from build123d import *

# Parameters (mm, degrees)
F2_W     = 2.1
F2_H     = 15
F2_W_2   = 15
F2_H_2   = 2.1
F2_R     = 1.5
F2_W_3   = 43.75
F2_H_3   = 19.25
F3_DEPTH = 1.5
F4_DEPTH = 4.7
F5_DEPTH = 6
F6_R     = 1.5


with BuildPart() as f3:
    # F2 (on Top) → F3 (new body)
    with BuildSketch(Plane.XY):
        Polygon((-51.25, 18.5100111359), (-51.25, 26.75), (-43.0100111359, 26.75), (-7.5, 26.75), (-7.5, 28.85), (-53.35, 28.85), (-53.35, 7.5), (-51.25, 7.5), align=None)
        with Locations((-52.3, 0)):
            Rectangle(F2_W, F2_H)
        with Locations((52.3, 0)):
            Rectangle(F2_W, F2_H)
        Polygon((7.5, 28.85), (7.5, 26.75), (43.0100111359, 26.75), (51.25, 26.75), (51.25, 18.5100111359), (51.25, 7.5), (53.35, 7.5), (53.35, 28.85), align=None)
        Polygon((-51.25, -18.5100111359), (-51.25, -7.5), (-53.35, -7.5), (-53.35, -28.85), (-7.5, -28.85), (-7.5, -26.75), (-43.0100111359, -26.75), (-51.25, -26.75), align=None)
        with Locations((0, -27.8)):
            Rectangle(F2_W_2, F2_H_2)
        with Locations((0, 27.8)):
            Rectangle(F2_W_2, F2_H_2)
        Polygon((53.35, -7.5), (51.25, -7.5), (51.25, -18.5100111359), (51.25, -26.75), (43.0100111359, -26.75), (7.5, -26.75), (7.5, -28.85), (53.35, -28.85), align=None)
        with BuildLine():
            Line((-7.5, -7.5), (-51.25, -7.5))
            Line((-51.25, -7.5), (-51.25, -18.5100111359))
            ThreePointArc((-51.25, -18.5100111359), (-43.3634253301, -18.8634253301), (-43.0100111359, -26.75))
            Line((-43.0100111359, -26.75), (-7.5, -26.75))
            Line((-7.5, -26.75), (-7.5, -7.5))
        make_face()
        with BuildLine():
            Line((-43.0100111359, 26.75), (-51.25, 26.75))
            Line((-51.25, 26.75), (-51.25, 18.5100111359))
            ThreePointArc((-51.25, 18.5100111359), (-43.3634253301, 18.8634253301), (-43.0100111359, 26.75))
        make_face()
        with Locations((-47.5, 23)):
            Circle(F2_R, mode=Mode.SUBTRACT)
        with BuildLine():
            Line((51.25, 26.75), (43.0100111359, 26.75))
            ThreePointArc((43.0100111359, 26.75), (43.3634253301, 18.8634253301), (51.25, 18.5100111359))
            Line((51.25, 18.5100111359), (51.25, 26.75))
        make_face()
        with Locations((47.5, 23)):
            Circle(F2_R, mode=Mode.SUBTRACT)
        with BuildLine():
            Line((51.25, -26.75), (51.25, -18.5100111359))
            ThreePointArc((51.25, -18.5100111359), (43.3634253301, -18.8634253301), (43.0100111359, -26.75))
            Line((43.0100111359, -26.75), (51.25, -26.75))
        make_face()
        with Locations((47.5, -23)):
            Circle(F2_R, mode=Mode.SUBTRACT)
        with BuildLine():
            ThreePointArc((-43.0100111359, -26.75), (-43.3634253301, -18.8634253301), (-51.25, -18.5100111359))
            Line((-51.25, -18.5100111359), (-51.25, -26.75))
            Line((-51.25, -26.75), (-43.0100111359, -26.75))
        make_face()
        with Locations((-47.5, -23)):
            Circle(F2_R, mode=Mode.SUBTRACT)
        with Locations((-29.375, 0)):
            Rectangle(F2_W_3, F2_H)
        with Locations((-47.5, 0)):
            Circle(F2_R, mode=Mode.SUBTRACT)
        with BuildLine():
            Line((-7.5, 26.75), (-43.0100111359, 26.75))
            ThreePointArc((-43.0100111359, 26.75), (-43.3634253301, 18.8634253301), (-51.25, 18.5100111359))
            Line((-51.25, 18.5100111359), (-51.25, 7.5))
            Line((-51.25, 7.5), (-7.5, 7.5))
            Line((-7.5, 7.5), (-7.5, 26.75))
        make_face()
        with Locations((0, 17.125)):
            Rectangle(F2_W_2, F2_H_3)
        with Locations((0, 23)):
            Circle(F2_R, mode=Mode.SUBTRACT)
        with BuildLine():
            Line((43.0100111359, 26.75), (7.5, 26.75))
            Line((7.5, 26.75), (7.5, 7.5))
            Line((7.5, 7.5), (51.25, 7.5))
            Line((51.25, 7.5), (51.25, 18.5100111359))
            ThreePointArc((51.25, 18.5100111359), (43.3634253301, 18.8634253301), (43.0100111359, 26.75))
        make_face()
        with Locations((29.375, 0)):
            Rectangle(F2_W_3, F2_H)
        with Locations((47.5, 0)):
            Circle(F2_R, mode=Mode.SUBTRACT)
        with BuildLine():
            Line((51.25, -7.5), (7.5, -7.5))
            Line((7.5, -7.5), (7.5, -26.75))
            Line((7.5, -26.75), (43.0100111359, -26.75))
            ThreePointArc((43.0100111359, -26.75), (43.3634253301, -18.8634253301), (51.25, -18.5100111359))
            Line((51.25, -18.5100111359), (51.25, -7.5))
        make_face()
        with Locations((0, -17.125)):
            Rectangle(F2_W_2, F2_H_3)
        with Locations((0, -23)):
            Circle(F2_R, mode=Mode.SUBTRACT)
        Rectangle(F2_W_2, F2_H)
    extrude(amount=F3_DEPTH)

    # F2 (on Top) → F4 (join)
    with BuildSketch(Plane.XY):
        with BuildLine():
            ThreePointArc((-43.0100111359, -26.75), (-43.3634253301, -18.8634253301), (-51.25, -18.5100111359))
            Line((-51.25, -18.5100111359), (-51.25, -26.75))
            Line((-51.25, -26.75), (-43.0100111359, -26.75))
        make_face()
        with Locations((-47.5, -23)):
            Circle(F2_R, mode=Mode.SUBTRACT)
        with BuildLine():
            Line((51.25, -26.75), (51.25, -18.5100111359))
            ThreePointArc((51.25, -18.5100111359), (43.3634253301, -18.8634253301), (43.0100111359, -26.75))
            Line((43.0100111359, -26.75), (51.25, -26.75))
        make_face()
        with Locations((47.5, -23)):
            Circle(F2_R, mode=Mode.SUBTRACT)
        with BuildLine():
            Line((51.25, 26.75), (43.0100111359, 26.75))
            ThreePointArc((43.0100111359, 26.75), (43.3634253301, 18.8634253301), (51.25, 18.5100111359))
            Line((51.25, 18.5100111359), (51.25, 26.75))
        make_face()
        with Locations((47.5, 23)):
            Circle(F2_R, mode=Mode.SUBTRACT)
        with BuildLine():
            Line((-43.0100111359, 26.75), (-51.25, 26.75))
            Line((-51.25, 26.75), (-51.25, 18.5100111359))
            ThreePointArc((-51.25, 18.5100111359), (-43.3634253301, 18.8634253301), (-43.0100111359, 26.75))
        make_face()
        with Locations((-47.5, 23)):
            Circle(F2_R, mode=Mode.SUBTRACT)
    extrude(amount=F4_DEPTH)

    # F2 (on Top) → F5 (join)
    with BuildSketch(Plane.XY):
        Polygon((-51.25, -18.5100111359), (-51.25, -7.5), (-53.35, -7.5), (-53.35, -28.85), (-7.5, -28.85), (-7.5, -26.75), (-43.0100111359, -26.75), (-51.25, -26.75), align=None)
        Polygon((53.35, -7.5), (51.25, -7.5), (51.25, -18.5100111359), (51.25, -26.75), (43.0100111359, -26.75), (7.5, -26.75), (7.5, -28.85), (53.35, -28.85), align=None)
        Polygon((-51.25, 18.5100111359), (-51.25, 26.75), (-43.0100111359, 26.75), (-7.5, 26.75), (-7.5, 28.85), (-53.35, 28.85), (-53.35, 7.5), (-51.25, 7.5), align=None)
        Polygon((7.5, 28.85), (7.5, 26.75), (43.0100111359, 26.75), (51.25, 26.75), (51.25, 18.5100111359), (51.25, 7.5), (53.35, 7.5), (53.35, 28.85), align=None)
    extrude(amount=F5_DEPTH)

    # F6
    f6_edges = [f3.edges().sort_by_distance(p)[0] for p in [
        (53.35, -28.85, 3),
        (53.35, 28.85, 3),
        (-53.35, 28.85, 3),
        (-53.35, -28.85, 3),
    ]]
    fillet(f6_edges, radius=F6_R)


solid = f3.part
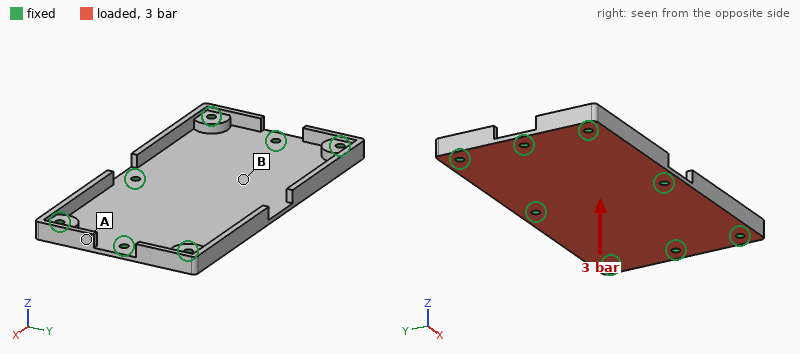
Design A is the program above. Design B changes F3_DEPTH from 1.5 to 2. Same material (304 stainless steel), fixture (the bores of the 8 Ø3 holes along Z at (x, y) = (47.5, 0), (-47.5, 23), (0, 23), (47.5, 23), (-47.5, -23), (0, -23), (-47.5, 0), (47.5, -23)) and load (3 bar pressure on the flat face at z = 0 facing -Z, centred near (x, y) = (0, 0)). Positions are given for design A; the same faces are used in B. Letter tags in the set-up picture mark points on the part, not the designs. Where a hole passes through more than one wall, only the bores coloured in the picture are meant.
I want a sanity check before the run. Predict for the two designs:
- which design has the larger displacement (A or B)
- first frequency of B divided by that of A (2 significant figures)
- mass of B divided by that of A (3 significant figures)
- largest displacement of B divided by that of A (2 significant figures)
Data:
A
1.3
1.21
0.45
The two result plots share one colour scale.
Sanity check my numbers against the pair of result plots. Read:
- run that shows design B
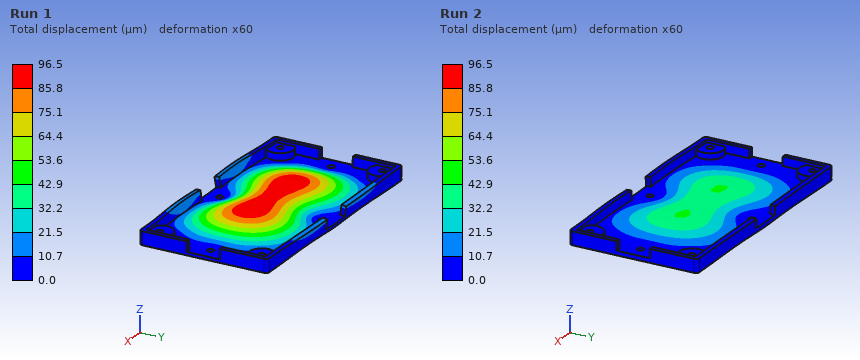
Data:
Run 2
